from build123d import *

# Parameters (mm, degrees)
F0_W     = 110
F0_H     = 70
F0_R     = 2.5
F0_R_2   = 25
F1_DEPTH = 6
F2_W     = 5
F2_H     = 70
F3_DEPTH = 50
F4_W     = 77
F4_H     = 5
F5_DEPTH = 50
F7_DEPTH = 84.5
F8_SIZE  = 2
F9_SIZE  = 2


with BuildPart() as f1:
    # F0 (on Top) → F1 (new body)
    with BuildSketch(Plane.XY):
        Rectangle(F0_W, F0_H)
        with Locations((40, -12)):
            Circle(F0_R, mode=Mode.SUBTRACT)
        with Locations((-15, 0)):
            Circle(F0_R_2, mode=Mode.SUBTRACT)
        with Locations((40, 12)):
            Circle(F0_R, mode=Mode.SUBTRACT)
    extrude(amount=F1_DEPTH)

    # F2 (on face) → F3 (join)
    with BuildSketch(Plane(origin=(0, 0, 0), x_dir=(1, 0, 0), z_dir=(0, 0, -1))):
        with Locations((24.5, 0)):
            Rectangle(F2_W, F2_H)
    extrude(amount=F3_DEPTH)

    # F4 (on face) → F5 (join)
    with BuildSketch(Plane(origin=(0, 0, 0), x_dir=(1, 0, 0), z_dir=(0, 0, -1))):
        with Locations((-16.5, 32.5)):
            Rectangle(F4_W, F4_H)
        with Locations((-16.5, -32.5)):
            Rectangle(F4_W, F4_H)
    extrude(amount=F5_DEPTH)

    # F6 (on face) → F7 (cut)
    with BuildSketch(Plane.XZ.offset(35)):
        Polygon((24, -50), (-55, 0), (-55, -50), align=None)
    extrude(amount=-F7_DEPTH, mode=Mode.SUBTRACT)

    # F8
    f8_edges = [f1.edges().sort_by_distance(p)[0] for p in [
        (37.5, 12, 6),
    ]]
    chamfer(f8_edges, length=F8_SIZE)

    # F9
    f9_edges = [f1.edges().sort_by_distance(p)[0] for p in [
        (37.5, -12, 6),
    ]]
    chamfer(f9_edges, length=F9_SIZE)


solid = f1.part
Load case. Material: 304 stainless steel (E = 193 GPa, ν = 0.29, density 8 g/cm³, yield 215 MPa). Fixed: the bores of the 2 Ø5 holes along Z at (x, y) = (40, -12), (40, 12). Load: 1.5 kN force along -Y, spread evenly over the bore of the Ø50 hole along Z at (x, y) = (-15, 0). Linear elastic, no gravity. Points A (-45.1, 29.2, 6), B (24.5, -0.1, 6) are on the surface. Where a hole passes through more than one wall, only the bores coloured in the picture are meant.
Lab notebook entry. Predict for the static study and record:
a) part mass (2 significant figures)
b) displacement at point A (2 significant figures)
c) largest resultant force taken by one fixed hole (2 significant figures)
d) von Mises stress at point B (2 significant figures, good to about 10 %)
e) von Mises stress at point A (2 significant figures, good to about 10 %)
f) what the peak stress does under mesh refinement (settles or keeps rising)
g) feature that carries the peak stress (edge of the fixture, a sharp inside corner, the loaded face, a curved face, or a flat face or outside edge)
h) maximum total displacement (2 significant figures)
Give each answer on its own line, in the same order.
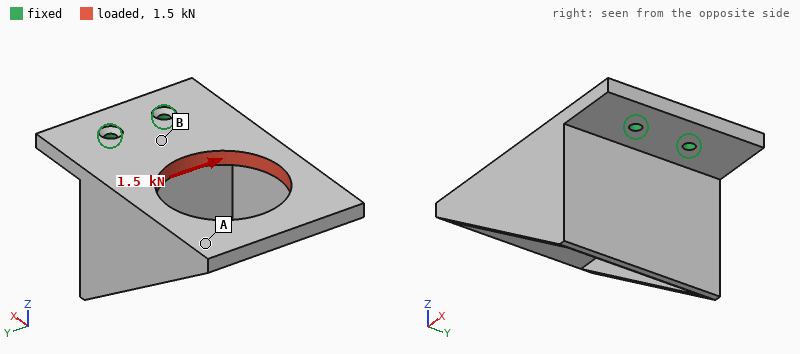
560 g
37 µm
3.1 kN
28 MPa
6.3 MPa
keeps rising
edge of the fixture
40 µm
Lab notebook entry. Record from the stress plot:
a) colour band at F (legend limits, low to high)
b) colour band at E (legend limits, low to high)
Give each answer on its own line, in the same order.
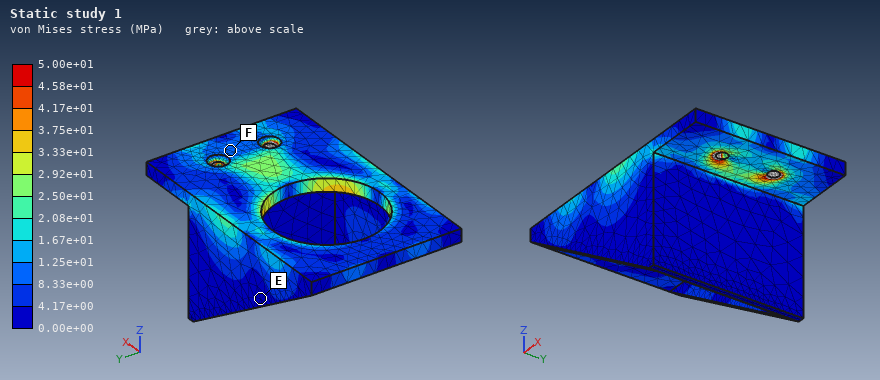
8.33e+00 to 1.25e+01 MPa
0.00e+00 to 4.17e+00 MPa
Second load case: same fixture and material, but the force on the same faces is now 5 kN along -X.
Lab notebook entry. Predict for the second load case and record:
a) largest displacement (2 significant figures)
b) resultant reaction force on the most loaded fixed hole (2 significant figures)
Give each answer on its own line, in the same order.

32 µm
2.5 kN
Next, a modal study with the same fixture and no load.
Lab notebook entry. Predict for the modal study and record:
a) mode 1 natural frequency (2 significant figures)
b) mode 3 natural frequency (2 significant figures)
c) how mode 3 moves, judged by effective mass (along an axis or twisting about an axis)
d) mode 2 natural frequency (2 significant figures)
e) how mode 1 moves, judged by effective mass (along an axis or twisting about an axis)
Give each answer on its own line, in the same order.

490 Hz
2000 Hz
along Y
1200 Hz
along Z
